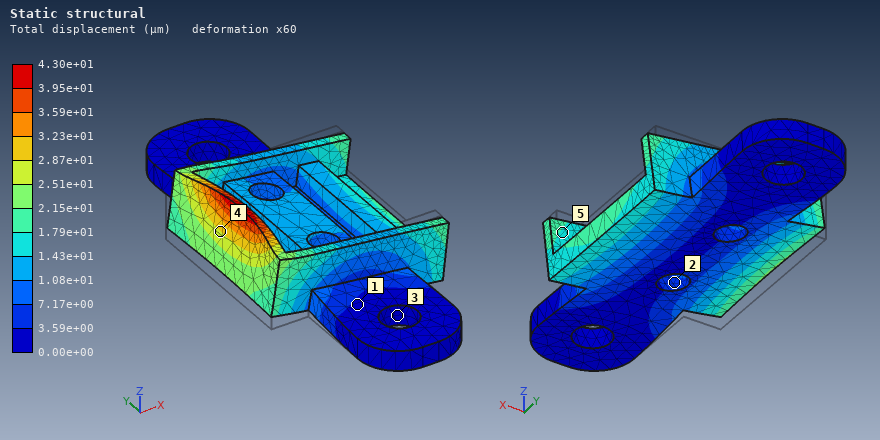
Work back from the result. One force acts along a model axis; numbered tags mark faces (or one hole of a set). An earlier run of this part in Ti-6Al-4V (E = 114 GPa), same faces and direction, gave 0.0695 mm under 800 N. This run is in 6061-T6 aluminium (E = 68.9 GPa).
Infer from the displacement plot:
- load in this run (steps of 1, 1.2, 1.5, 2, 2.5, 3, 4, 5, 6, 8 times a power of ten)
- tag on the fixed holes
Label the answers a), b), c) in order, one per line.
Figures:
a) 300 N
b) 3
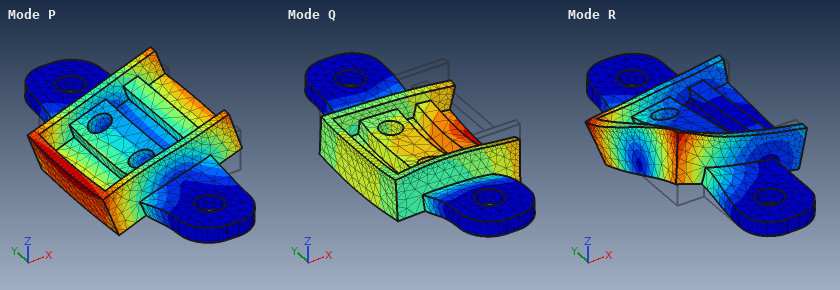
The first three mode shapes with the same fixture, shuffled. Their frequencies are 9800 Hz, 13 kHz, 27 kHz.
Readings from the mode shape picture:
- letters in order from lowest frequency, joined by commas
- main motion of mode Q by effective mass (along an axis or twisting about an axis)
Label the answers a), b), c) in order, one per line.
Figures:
a) P, Q, R
b) along Z
